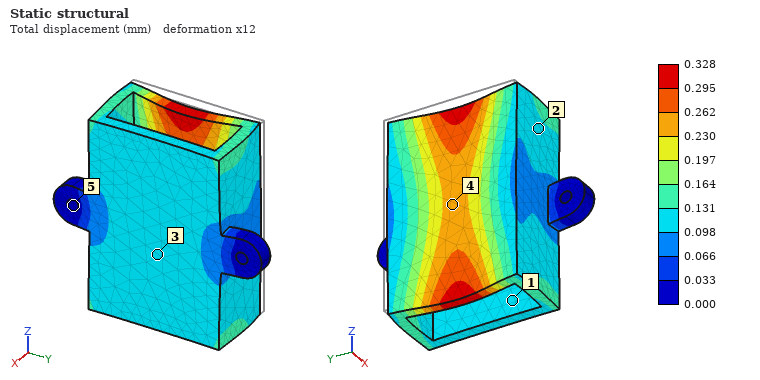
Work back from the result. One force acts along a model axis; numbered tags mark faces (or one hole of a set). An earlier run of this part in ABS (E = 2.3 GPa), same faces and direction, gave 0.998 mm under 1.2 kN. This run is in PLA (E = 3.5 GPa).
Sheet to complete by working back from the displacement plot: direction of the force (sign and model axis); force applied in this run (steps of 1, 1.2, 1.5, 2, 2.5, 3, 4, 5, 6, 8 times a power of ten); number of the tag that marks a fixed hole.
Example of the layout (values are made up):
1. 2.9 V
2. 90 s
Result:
1. +X
2. 600 N
3. 5
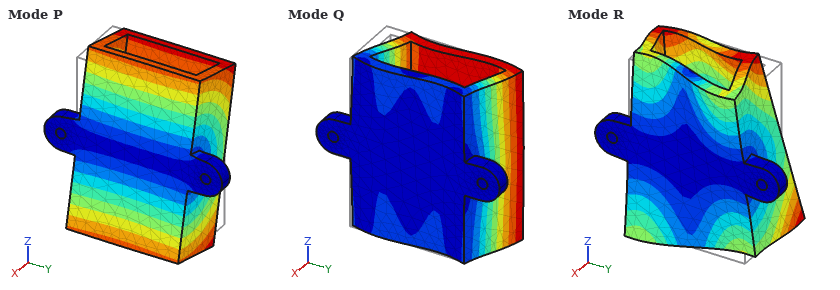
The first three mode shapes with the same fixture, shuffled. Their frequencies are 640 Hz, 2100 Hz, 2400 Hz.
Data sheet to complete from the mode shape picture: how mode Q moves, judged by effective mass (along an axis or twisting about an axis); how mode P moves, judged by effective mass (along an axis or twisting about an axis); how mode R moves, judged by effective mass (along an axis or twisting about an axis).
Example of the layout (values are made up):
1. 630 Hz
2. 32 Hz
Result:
1. along Y
2. along Z
3. twisting about X
